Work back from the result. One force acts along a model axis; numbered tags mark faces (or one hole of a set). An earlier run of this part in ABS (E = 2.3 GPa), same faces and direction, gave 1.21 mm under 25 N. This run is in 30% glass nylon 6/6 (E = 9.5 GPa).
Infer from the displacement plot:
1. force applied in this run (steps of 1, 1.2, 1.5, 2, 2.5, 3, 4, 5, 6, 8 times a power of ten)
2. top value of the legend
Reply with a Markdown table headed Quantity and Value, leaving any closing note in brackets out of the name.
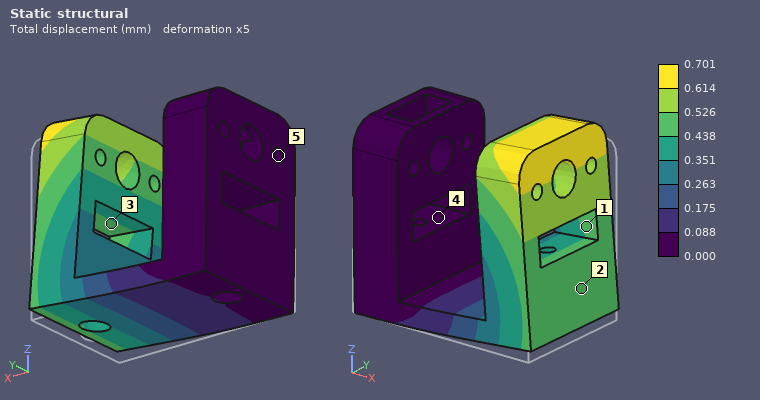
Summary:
| Quantity | Value |
|---|---|
| force applied in this run | 60 N |
| top value of the legend | 0.701 mm |
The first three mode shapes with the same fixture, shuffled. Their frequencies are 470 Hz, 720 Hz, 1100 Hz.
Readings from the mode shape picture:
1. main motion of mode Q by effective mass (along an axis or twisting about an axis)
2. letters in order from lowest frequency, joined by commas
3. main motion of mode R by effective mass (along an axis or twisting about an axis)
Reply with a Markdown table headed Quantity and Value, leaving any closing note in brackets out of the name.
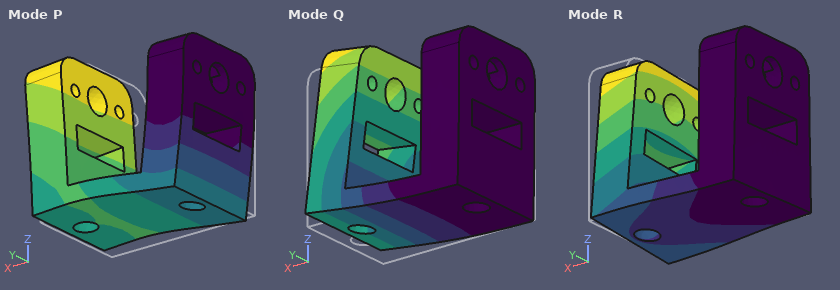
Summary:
| Quantity | Value |
|---|---|
| main motion of mode Q by effective mass | along Z |
| letters in order from lowest frequency, joined by commas | Q, R, P |
| main motion of mode R by effective mass | along Y |
